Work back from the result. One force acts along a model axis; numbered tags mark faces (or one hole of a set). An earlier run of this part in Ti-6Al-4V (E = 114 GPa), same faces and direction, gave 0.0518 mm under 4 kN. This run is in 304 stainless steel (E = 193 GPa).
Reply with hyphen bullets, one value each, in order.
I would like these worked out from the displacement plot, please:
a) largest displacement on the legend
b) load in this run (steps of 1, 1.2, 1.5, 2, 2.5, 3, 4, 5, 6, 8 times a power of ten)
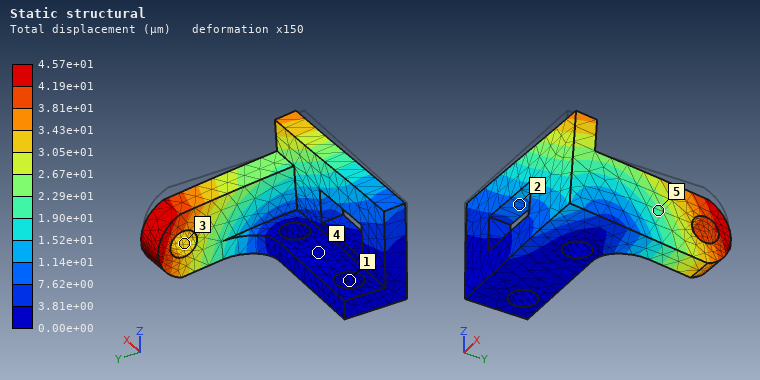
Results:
- 4.57e+01 µm
- 6 kN
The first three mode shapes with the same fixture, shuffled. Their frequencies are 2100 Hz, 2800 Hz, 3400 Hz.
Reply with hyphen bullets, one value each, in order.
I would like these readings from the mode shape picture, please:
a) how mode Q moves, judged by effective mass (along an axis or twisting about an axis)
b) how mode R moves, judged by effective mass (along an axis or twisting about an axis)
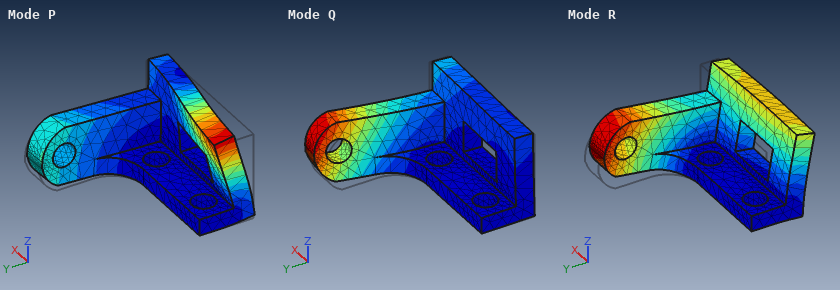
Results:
- along X
- along Y
